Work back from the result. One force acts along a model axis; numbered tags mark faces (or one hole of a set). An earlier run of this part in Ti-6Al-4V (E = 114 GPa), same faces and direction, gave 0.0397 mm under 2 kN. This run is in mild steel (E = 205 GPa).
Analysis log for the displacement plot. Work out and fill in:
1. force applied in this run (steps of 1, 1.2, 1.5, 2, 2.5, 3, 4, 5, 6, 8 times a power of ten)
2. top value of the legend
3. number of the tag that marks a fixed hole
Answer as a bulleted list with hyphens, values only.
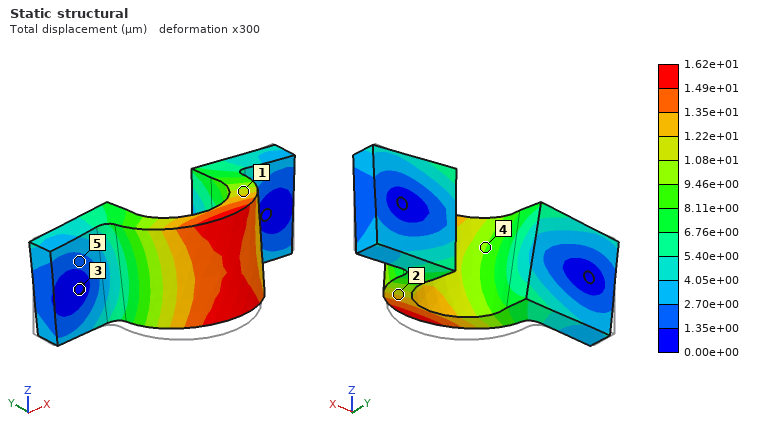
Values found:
- 1.5 kN
- 1.62e+01 µm
- 3
